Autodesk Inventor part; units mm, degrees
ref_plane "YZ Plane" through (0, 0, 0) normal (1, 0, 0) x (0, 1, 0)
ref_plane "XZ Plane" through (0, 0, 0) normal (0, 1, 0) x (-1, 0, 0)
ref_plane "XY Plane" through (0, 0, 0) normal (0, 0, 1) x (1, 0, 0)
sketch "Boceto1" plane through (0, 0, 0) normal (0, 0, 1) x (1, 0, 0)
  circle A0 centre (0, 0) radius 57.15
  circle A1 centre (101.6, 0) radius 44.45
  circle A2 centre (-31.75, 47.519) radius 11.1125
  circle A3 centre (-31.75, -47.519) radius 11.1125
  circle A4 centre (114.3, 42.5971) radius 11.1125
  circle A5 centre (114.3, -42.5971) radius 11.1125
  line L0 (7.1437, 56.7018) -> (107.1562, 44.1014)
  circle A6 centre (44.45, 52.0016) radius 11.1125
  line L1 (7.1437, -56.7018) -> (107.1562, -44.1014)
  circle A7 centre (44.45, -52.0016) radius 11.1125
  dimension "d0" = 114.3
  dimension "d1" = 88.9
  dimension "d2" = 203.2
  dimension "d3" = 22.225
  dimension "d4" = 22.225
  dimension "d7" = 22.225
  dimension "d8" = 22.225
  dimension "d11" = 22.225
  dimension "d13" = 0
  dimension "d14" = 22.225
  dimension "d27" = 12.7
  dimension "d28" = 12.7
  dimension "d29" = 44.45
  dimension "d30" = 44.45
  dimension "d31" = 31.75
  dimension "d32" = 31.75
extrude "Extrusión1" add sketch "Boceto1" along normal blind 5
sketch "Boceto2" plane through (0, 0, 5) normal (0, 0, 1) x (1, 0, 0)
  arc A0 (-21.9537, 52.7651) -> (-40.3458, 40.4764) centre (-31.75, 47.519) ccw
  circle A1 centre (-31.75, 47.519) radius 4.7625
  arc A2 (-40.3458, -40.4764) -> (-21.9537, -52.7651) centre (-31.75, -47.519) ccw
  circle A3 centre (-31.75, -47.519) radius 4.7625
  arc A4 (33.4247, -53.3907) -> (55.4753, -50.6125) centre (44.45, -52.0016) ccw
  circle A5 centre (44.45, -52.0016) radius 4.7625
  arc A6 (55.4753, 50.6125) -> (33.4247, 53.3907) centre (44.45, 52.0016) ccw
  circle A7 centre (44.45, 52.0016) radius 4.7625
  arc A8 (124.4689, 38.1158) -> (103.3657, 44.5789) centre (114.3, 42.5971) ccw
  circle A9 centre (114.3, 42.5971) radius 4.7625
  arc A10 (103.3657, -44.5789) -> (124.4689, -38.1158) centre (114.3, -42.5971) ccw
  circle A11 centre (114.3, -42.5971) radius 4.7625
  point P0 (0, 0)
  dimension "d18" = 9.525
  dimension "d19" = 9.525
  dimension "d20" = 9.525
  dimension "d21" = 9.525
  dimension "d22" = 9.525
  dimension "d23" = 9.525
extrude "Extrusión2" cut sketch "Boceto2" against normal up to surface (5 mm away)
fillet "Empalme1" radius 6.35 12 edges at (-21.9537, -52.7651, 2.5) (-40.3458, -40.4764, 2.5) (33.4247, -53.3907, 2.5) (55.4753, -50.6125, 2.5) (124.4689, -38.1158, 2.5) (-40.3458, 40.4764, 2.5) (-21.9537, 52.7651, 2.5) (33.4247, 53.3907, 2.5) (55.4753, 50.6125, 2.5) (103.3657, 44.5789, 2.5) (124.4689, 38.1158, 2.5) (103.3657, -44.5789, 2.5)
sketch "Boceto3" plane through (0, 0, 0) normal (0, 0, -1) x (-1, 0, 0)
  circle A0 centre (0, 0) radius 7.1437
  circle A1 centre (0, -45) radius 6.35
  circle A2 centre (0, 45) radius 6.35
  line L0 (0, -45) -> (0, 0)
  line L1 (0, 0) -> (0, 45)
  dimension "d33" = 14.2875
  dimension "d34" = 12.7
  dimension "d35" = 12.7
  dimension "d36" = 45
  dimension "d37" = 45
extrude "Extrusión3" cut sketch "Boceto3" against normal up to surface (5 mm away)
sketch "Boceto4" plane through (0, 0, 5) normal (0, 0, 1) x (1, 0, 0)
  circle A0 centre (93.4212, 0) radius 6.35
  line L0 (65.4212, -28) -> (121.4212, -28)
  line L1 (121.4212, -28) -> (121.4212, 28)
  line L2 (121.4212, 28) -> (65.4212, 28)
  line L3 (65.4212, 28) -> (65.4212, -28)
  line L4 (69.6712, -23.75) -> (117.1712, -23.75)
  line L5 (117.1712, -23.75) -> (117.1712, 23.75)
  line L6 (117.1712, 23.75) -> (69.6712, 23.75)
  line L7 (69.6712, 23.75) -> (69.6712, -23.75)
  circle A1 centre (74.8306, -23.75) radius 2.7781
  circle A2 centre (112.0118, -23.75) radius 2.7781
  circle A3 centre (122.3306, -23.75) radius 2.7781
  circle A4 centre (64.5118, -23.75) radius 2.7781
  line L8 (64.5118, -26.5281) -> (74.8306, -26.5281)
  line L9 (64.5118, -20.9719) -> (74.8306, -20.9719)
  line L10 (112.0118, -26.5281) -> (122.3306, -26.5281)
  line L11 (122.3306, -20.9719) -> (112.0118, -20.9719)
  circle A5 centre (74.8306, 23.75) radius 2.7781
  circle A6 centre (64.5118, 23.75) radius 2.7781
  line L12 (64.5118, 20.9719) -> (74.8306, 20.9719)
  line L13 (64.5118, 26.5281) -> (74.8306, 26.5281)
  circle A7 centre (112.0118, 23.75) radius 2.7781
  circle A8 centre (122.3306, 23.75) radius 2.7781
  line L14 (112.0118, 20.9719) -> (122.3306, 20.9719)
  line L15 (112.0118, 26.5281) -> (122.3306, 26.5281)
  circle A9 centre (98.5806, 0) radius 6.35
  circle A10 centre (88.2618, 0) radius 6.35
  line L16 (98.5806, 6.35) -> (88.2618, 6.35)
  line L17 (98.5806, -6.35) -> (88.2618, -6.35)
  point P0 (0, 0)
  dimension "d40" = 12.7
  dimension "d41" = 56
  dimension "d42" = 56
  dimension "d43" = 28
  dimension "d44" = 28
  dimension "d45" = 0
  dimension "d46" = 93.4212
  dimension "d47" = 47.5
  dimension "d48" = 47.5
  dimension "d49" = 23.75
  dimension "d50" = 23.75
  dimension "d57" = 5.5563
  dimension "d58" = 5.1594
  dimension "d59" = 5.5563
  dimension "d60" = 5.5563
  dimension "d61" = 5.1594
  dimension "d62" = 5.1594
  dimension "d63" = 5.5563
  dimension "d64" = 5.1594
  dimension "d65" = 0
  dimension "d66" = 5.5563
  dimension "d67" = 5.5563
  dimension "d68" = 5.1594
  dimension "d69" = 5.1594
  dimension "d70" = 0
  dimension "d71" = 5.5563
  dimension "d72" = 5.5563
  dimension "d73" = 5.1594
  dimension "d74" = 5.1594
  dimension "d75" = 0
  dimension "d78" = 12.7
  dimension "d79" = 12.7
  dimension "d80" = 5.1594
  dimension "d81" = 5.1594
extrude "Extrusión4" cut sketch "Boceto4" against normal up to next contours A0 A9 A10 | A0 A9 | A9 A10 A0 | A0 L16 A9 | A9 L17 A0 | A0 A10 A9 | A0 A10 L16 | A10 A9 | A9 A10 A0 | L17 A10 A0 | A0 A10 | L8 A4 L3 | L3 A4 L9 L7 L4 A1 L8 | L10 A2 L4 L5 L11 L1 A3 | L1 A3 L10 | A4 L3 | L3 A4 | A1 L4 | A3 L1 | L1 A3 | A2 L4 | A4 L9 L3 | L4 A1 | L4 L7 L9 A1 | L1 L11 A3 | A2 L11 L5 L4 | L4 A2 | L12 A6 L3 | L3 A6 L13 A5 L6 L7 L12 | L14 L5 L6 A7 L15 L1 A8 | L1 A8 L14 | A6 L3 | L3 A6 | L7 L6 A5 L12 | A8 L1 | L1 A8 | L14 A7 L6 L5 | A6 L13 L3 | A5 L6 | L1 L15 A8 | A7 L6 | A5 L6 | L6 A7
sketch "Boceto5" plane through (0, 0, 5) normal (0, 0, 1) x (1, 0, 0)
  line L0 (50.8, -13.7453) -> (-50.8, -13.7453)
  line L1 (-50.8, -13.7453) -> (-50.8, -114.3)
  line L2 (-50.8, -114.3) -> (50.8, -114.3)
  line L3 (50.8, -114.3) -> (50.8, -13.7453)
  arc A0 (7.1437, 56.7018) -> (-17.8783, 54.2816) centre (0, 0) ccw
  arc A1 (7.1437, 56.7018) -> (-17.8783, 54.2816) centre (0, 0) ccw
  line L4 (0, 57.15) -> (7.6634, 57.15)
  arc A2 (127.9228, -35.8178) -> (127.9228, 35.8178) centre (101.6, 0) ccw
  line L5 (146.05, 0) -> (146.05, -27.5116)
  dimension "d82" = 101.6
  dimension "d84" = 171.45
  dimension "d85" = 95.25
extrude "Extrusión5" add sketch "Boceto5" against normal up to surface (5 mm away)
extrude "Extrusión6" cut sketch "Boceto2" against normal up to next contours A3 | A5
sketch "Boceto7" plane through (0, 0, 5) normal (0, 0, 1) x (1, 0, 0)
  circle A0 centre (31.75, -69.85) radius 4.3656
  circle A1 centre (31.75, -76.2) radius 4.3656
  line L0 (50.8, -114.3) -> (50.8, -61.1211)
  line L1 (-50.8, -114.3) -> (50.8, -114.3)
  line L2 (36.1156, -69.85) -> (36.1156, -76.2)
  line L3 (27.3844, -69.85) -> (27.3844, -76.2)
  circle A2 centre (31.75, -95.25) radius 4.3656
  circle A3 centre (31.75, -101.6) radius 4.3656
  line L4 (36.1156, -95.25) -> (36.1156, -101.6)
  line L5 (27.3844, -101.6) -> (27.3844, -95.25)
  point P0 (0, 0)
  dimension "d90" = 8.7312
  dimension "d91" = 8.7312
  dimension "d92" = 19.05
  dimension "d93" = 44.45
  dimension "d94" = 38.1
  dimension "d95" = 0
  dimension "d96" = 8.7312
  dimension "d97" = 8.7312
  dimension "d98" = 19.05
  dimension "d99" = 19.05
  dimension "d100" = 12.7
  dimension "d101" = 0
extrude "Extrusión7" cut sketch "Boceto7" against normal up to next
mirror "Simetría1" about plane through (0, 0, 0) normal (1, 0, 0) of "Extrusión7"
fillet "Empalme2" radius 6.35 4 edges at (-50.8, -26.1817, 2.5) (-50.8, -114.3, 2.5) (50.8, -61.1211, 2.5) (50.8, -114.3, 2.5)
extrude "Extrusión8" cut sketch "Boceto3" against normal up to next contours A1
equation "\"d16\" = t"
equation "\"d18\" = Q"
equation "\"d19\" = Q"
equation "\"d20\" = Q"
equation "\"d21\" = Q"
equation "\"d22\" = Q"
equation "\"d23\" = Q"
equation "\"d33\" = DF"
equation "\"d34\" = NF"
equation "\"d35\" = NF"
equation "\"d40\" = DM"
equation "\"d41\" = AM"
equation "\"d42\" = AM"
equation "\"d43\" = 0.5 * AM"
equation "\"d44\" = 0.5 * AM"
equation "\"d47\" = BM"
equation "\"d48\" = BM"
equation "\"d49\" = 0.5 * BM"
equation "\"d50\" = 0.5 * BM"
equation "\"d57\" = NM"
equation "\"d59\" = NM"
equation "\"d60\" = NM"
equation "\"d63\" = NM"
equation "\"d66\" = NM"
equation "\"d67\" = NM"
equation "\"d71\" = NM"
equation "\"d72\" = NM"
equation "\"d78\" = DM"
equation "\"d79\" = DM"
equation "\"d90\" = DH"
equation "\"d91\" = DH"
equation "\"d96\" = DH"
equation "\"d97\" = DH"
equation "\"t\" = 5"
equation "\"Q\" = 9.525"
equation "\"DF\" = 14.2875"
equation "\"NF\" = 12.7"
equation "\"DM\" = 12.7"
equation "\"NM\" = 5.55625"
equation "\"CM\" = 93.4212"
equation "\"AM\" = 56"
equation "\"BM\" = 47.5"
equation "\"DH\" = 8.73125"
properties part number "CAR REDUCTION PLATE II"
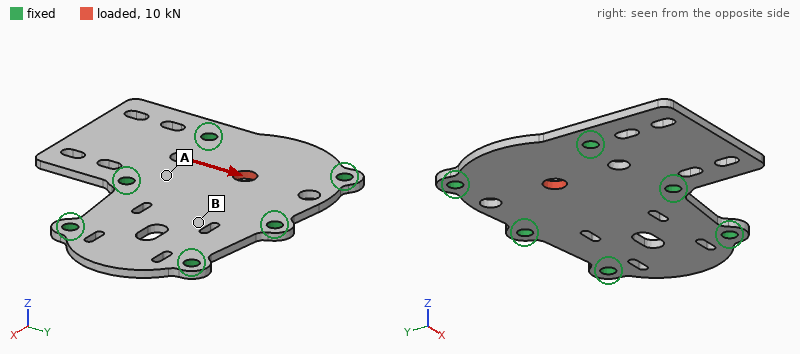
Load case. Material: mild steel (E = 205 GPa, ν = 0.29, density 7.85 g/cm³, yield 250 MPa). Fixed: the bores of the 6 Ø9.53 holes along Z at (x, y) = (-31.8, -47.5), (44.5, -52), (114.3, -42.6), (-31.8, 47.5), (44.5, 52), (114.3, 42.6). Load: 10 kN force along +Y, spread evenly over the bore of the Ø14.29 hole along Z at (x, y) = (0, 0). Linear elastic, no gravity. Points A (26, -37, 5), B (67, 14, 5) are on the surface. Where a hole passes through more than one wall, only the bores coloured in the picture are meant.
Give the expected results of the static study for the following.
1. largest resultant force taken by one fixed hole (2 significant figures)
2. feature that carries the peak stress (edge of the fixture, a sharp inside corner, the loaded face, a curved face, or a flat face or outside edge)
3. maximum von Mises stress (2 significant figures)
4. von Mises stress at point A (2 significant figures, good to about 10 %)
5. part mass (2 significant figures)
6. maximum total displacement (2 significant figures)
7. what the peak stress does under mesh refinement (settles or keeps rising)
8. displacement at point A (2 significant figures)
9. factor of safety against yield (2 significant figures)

3.2 kN
the loaded face
78 MPa
14 MPa
940 g
7.1 µm
settles
2.0 µm
3.2
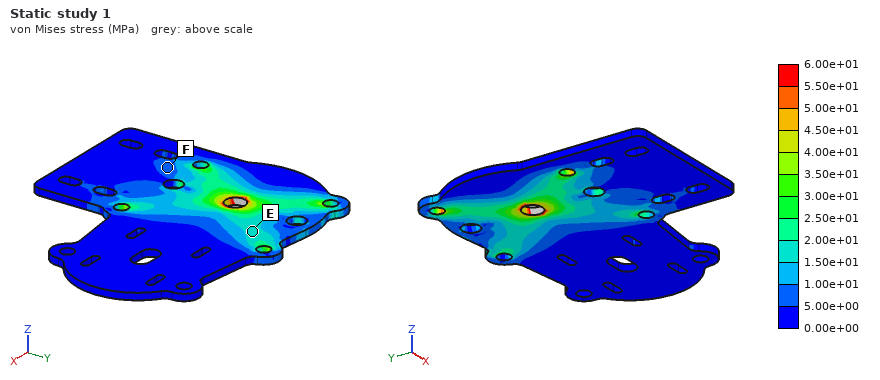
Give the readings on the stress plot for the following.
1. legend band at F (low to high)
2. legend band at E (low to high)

5.00e+00 to 1.00e+01 MPa
1.50e+01 to 2.00e+01 MPa
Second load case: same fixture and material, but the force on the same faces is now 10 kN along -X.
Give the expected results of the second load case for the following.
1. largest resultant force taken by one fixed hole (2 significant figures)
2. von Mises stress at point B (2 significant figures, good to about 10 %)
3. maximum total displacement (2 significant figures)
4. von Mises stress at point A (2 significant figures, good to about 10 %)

2.6 kN
8.8 MPa
8.4 µm
15 MPa
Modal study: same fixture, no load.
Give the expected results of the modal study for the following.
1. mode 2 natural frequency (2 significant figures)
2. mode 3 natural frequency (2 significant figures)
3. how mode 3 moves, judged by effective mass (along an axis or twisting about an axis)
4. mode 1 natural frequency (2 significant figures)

1900 Hz
2400 Hz
along Z
940 Hz
